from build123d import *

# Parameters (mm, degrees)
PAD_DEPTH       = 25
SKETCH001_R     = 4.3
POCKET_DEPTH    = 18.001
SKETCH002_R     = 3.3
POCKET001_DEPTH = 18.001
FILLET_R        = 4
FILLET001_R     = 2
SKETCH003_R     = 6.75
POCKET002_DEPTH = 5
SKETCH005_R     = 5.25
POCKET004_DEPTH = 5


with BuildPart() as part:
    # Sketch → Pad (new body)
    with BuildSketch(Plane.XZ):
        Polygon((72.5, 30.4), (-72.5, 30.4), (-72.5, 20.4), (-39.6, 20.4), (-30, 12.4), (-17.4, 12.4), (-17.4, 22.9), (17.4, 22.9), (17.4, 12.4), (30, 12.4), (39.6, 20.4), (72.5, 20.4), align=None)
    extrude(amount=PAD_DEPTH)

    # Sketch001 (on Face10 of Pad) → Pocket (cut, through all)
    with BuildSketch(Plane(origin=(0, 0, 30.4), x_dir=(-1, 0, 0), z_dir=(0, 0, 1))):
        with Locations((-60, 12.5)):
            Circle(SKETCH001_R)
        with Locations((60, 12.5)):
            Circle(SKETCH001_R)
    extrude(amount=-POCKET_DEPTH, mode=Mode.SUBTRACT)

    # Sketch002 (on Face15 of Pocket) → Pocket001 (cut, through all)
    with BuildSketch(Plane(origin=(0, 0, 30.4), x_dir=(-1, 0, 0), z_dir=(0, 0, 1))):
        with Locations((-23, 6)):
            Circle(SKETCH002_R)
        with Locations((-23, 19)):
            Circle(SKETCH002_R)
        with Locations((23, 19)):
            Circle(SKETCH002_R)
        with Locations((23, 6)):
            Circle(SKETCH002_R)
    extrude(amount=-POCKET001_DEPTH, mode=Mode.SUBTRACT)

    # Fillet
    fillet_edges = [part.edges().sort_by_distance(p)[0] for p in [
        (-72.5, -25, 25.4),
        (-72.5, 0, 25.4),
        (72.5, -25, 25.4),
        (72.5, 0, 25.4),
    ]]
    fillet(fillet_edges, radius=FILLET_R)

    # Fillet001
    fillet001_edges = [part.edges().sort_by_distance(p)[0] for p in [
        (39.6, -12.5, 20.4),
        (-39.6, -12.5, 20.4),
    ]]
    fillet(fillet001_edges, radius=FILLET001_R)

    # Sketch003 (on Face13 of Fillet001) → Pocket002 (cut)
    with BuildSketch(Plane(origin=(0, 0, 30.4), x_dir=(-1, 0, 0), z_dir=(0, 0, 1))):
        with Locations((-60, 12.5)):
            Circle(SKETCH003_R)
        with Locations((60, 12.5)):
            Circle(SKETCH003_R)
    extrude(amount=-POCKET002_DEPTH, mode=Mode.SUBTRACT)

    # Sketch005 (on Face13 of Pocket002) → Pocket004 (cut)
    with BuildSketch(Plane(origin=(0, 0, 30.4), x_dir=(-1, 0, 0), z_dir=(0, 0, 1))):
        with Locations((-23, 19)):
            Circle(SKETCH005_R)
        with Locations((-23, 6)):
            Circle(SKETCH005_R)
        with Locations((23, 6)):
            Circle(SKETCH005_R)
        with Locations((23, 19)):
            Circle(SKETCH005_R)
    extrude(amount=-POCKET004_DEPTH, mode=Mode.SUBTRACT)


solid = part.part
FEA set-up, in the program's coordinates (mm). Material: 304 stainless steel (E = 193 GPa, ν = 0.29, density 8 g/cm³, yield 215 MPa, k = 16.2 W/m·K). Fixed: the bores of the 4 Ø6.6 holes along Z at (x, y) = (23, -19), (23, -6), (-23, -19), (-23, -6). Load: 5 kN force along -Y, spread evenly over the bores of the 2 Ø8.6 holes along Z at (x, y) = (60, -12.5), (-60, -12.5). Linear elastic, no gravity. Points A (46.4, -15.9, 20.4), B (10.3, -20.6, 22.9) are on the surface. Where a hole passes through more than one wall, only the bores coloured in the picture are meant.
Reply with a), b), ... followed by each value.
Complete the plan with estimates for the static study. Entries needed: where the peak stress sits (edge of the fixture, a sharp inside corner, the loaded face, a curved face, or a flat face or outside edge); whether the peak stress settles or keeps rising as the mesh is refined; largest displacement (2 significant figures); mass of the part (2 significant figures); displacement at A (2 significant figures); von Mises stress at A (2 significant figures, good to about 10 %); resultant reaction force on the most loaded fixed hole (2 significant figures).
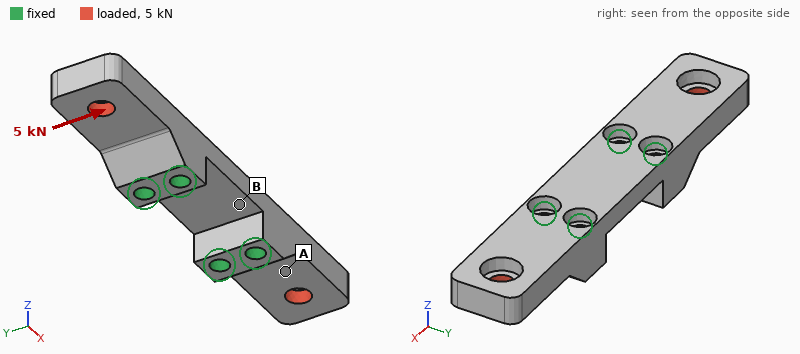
a) edge of the fixture
b) keeps rising
c) 34 µm
d) 280 g
e) 11 µm
f) 44 MPa
g) 5.2 kN
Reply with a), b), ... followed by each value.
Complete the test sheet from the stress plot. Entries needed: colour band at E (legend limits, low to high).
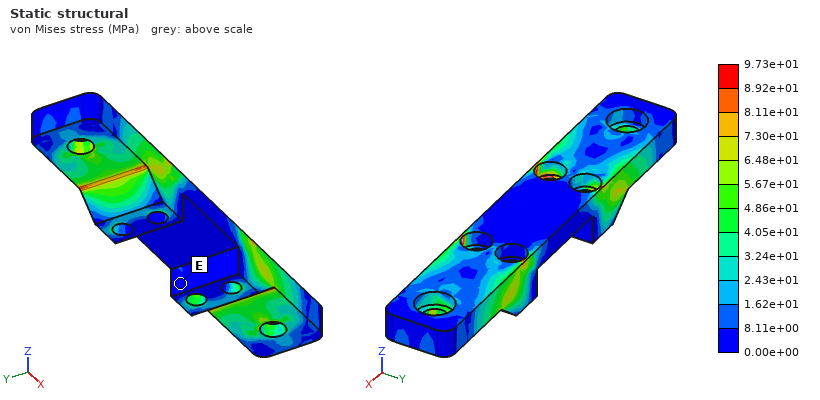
a) 0.00e+00 to 8.11e+00 MPa
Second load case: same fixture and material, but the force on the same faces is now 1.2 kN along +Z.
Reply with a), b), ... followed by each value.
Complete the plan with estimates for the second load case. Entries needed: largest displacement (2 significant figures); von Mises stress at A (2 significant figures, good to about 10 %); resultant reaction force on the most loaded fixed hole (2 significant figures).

a) 24 µm
b) 19 MPa
c) 330 N
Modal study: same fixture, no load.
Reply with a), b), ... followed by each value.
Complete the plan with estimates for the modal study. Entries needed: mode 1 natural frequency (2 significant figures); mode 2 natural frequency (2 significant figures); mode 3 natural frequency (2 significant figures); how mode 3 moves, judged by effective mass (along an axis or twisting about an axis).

a) 4600 Hz
b) 4600 Hz
c) 7700 Hz
d) along Y
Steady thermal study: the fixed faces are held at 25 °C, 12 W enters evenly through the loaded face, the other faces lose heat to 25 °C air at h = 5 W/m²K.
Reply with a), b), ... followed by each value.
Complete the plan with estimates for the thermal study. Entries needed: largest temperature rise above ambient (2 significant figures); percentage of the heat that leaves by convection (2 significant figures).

a) 59 K
b) 9.3 %
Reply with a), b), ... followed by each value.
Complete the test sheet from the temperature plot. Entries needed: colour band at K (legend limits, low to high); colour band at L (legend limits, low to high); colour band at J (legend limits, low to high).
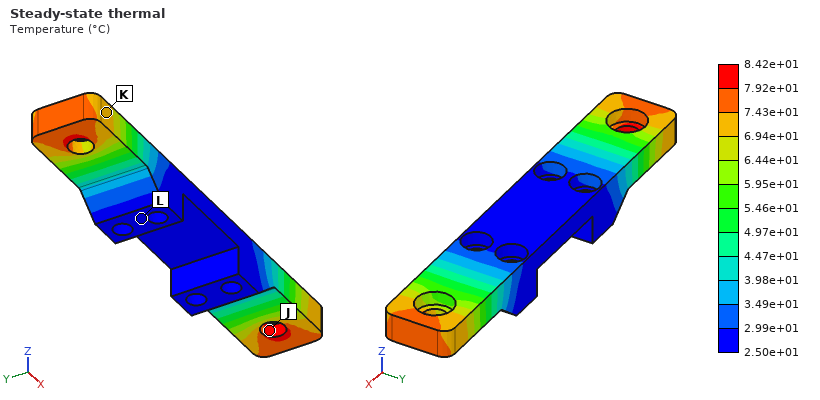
a) 6.94e+01 to 7.43e+01 °C
b) 2.50e+01 to 2.99e+01 °C
c) 7.92e+01 to 8.42e+01 °C
